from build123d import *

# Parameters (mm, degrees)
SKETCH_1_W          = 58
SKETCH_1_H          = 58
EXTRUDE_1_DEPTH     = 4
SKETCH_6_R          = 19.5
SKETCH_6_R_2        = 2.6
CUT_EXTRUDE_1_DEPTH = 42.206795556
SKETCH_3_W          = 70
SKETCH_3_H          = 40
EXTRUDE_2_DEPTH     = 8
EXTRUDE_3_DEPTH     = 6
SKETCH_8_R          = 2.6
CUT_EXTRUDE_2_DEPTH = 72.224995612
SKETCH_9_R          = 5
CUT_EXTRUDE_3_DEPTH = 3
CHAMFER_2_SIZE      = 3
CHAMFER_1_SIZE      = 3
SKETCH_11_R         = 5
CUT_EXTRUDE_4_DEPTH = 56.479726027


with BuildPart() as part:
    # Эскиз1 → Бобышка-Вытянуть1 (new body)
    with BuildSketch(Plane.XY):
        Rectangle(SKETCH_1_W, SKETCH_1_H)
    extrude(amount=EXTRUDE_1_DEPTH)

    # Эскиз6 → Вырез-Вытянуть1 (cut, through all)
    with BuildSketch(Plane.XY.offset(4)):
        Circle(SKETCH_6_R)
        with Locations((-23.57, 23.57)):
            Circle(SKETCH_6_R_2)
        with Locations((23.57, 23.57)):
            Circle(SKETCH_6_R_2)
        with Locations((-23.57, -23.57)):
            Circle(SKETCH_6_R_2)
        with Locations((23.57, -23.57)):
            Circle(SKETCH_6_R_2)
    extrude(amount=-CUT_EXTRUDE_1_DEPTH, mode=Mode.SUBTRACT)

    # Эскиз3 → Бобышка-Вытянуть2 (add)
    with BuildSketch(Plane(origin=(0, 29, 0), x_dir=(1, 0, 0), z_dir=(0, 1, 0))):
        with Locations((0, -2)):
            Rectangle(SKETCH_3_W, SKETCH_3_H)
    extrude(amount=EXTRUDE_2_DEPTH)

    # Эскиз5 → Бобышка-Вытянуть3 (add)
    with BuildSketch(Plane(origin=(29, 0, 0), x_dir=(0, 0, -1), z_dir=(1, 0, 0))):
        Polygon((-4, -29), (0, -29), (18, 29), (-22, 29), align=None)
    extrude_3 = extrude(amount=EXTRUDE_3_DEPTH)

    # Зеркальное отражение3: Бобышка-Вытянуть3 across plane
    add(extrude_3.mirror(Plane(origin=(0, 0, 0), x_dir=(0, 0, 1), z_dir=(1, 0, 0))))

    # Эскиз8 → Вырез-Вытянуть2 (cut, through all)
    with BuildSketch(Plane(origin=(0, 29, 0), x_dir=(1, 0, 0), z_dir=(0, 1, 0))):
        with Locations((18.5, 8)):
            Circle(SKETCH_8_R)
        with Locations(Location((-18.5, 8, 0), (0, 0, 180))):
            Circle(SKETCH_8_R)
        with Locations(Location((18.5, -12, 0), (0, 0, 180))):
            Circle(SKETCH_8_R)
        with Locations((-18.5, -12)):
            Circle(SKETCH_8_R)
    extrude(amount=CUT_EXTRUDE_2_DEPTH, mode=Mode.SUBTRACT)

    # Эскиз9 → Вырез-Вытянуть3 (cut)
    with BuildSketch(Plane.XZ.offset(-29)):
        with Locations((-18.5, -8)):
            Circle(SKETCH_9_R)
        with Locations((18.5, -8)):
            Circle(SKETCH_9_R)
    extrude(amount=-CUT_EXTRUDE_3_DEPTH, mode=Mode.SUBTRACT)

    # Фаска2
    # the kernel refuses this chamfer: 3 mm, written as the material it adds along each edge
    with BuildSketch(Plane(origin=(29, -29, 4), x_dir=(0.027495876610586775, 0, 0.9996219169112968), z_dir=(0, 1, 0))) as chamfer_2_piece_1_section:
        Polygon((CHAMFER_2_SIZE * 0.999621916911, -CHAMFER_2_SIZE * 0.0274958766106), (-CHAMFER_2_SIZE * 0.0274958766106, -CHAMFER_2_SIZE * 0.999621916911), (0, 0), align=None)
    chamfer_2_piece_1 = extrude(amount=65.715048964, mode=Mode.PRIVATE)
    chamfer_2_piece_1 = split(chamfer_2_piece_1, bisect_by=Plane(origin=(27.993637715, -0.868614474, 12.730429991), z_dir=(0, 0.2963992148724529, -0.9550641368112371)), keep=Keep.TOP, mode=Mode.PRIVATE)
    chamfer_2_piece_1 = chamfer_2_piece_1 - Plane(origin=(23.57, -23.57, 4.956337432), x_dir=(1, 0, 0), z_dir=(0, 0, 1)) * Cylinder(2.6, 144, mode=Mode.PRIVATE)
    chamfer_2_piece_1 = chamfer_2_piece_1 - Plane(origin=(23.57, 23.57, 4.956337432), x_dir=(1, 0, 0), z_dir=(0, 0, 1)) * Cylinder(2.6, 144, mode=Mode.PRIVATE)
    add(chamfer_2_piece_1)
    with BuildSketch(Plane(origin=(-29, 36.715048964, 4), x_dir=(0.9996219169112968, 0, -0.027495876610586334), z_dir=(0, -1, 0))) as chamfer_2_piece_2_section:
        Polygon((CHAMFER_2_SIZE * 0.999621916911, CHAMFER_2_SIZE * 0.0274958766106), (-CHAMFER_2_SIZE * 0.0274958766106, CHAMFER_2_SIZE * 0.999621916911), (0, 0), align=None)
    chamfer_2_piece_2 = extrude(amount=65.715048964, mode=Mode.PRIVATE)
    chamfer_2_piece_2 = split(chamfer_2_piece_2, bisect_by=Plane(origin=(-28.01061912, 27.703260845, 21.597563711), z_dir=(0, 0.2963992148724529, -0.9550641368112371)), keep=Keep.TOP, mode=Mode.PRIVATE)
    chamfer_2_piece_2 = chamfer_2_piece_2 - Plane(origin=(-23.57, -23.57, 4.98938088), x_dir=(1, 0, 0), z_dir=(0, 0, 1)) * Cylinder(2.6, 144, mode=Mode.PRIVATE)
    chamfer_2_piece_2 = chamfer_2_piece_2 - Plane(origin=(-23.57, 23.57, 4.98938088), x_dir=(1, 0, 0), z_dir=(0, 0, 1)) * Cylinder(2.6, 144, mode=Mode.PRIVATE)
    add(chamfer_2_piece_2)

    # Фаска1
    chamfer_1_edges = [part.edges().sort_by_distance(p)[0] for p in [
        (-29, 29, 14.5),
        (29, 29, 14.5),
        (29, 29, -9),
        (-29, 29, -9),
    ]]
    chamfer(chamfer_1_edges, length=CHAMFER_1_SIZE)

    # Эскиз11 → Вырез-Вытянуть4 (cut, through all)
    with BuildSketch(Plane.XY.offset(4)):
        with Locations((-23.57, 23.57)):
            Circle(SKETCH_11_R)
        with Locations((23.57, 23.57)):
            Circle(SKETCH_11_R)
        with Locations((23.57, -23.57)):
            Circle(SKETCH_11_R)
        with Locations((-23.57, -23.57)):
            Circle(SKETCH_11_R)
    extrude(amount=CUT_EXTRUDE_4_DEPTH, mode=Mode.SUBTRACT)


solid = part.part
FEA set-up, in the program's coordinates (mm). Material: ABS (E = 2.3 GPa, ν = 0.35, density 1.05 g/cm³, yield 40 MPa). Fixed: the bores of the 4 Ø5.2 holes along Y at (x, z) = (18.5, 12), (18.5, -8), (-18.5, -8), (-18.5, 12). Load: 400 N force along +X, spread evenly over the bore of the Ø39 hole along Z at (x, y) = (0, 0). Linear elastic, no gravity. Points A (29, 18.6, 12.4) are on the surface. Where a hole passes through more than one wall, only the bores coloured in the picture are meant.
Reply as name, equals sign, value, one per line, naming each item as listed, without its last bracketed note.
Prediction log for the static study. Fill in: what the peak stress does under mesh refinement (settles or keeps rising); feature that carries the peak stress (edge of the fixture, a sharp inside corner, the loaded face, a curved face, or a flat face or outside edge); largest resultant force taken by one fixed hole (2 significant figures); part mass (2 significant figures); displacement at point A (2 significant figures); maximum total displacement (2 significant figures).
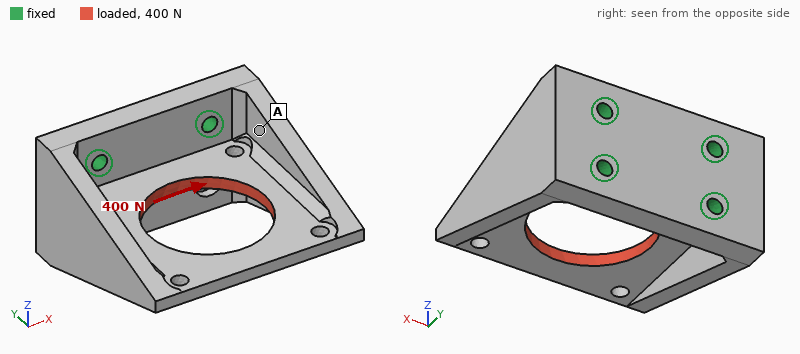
what the peak stress does under mesh refinement = keeps rising
feature that carries the peak stress = edge of the fixture
largest resultant force taken by one fixed hole = 200 N
part mass = 48 g
displacement at point A = 0.079 mm
maximum total displacement = 0.37 mm
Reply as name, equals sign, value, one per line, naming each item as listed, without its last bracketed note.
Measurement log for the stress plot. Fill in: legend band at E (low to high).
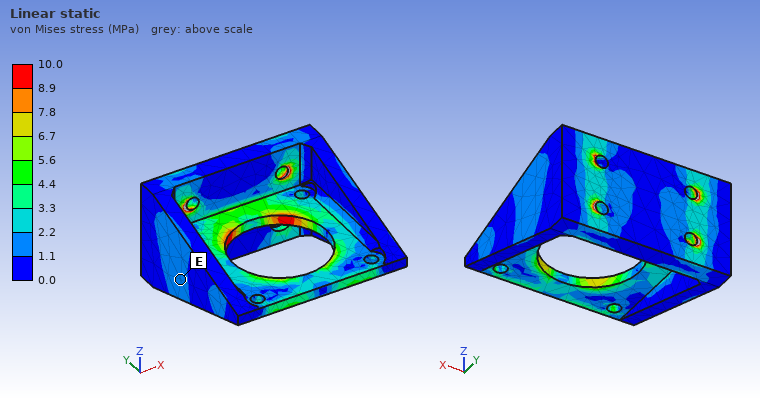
legend band at E = 1.1 to 2.2 MPa
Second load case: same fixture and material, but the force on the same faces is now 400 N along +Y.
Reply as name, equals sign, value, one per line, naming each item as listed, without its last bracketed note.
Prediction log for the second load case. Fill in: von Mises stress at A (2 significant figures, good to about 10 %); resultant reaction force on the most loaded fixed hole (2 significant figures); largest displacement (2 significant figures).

von Mises stress at A = 0.84 MPa
resultant reaction force on the most loaded fixed hole = 110 N
largest displacement = 0.11 mm
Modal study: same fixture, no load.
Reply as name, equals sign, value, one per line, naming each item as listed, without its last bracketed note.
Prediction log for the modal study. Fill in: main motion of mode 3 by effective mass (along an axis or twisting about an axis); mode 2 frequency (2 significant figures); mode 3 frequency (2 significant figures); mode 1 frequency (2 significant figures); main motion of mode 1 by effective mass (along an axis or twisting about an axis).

main motion of mode 3 by effective mass = along X
mode 2 frequency = 1300 Hz
mode 3 frequency = 1400 Hz
mode 1 frequency = 960 Hz
main motion of mode 1 by effective mass = along Z
